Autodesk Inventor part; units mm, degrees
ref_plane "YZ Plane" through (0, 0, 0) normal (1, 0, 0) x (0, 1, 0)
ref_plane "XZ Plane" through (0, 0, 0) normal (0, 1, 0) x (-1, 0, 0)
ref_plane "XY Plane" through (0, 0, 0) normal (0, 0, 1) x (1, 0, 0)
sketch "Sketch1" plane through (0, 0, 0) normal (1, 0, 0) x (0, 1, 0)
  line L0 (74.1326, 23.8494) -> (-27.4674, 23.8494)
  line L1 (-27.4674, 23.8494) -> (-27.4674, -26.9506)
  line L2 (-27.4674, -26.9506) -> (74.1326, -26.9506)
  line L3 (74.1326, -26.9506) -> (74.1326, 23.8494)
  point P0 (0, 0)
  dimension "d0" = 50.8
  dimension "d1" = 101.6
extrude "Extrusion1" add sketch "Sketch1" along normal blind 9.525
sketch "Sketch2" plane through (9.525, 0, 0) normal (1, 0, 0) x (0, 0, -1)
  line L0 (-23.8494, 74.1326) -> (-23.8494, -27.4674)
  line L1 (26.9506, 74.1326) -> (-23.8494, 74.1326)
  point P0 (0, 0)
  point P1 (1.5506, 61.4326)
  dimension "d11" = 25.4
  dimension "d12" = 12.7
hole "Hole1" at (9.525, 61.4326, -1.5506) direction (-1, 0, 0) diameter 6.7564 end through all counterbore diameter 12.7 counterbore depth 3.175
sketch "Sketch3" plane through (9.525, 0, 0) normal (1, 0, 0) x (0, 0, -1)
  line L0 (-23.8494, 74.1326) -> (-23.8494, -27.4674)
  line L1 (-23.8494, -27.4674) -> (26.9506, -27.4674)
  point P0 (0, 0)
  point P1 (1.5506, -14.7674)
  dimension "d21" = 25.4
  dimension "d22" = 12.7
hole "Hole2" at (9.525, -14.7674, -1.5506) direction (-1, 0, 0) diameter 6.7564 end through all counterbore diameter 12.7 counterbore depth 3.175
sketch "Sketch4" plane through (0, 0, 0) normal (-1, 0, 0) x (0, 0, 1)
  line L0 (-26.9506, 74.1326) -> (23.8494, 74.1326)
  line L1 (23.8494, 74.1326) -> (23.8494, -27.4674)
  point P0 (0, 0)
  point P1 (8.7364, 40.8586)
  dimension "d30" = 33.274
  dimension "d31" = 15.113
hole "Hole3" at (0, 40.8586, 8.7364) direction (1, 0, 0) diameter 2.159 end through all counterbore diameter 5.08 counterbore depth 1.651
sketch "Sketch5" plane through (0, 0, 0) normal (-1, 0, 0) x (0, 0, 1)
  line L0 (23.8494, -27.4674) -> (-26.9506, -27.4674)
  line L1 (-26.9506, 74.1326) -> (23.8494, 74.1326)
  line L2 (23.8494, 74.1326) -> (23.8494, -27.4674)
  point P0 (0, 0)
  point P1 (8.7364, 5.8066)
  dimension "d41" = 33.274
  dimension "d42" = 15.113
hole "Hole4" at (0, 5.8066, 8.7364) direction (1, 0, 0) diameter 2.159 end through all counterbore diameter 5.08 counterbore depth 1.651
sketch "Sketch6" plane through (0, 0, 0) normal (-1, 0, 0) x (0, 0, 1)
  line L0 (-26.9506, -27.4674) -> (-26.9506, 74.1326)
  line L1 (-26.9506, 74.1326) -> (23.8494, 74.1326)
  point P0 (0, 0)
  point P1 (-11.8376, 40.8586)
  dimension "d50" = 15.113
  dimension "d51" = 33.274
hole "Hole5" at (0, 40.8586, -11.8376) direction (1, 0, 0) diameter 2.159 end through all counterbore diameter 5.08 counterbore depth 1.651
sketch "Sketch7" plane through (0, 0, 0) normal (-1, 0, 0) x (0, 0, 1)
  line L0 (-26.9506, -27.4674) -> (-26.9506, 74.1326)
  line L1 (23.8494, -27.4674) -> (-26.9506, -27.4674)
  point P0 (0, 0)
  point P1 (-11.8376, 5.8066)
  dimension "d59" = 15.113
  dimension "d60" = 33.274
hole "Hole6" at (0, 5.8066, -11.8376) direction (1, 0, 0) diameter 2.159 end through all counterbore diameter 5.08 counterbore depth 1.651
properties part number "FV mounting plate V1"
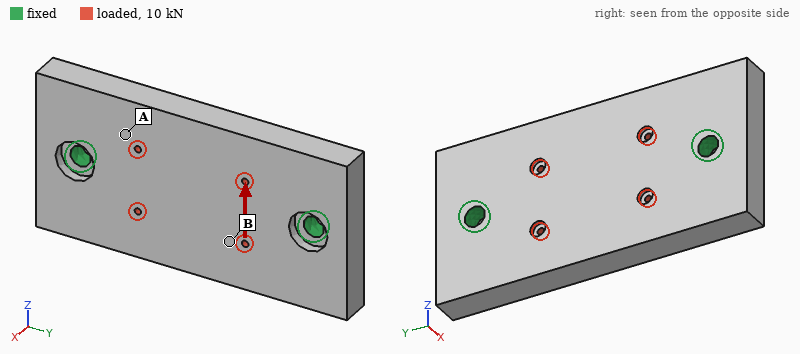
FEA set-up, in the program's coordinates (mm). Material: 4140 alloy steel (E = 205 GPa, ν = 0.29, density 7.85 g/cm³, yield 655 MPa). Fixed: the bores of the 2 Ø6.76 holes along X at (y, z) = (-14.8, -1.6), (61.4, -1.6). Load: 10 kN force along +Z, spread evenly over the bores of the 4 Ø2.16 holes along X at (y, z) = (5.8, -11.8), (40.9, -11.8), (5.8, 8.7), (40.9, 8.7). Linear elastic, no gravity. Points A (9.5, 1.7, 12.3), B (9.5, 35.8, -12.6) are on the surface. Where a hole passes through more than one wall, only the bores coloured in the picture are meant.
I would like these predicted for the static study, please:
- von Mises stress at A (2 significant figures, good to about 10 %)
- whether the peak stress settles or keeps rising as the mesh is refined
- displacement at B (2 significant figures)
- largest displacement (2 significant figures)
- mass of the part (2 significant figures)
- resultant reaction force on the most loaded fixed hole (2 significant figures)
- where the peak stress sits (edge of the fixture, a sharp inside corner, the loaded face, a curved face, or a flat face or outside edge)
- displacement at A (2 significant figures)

26 MPa
keeps rising
9.2 µm
13 µm
370 g
5.0 kN
edge of the fixture
8.4 µm
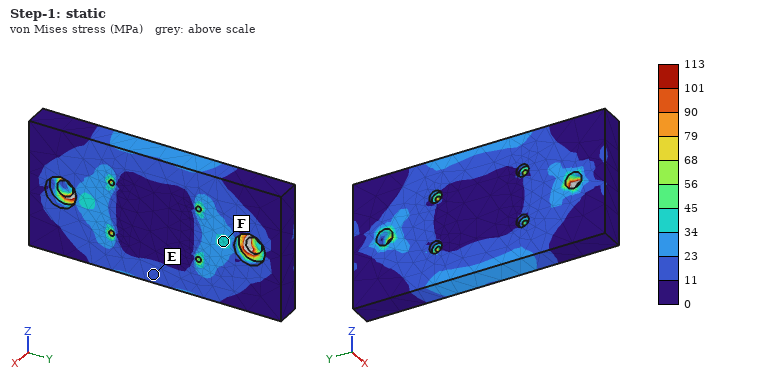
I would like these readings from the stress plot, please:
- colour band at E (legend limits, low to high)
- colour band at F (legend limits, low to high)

11 to 23 MPa
34 to 45 MPa
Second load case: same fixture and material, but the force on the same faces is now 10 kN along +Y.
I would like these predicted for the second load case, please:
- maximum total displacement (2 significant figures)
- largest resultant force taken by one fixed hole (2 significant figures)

3.3 µm
5.0 kN
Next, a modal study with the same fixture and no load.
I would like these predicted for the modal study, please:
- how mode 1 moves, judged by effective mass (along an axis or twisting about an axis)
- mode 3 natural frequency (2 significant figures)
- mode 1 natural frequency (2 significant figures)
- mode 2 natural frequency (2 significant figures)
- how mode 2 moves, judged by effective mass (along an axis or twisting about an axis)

twisting about Y
8700 Hz
4700 Hz
5400 Hz
along X
